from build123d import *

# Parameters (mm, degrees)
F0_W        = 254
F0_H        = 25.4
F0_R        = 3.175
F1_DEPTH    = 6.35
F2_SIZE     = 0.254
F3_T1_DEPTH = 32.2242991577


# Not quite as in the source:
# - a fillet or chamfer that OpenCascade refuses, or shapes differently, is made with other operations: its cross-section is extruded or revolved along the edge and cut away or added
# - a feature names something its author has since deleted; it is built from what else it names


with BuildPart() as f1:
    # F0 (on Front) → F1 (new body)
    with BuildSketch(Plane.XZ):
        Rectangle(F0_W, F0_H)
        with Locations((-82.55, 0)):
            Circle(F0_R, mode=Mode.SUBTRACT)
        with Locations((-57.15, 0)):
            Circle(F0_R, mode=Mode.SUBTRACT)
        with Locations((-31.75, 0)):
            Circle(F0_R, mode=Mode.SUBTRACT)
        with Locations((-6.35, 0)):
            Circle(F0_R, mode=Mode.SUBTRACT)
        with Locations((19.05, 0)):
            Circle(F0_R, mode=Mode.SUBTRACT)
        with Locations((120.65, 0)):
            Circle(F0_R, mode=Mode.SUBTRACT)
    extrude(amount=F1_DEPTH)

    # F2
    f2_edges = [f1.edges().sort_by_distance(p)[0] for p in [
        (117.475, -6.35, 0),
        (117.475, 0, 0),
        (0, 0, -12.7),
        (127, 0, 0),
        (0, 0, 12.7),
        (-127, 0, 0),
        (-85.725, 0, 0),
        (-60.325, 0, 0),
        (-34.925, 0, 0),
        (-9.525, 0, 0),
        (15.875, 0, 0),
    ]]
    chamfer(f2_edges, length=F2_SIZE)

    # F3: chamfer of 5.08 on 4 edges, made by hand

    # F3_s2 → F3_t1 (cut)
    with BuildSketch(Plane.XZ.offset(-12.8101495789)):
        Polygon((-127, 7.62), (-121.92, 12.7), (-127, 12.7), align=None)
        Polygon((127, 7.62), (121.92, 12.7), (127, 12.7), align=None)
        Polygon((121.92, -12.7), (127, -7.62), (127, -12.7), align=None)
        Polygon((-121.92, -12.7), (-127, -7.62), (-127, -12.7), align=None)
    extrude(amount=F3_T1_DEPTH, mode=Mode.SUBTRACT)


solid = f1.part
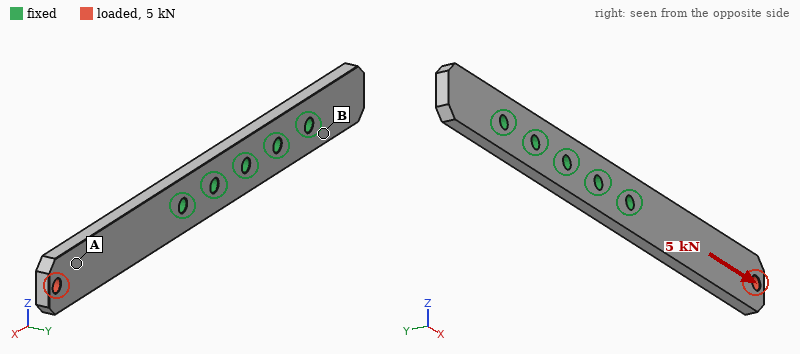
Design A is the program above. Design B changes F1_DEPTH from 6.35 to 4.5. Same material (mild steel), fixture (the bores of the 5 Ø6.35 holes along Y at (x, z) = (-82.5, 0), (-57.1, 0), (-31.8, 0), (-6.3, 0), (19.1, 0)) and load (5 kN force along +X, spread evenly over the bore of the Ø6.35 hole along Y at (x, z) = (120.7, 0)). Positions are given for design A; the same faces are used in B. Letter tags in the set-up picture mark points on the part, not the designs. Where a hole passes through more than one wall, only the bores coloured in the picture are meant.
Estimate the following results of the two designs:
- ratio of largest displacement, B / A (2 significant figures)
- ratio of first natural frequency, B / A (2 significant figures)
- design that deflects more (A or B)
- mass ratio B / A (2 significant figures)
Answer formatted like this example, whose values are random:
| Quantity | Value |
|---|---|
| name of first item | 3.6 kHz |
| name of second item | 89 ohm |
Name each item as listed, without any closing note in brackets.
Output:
| Quantity | Value |
|---|---|
| ratio of largest displacement, B / A | 1.4 |
| ratio of first natural frequency, B / A | 0.72 |
| design that deflects more | B |
| mass ratio B / A | 0.71 |
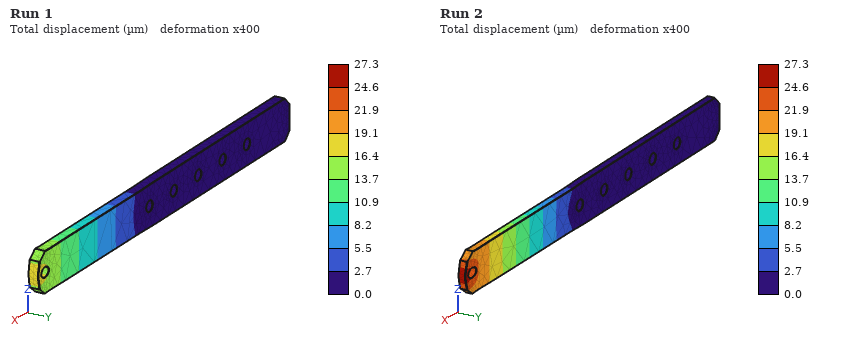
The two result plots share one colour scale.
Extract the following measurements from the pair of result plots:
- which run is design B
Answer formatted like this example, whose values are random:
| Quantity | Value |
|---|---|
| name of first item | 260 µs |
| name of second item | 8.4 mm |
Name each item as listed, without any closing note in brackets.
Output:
| Quantity | Value |
|---|---|
| which run is design B | Run 2 |
